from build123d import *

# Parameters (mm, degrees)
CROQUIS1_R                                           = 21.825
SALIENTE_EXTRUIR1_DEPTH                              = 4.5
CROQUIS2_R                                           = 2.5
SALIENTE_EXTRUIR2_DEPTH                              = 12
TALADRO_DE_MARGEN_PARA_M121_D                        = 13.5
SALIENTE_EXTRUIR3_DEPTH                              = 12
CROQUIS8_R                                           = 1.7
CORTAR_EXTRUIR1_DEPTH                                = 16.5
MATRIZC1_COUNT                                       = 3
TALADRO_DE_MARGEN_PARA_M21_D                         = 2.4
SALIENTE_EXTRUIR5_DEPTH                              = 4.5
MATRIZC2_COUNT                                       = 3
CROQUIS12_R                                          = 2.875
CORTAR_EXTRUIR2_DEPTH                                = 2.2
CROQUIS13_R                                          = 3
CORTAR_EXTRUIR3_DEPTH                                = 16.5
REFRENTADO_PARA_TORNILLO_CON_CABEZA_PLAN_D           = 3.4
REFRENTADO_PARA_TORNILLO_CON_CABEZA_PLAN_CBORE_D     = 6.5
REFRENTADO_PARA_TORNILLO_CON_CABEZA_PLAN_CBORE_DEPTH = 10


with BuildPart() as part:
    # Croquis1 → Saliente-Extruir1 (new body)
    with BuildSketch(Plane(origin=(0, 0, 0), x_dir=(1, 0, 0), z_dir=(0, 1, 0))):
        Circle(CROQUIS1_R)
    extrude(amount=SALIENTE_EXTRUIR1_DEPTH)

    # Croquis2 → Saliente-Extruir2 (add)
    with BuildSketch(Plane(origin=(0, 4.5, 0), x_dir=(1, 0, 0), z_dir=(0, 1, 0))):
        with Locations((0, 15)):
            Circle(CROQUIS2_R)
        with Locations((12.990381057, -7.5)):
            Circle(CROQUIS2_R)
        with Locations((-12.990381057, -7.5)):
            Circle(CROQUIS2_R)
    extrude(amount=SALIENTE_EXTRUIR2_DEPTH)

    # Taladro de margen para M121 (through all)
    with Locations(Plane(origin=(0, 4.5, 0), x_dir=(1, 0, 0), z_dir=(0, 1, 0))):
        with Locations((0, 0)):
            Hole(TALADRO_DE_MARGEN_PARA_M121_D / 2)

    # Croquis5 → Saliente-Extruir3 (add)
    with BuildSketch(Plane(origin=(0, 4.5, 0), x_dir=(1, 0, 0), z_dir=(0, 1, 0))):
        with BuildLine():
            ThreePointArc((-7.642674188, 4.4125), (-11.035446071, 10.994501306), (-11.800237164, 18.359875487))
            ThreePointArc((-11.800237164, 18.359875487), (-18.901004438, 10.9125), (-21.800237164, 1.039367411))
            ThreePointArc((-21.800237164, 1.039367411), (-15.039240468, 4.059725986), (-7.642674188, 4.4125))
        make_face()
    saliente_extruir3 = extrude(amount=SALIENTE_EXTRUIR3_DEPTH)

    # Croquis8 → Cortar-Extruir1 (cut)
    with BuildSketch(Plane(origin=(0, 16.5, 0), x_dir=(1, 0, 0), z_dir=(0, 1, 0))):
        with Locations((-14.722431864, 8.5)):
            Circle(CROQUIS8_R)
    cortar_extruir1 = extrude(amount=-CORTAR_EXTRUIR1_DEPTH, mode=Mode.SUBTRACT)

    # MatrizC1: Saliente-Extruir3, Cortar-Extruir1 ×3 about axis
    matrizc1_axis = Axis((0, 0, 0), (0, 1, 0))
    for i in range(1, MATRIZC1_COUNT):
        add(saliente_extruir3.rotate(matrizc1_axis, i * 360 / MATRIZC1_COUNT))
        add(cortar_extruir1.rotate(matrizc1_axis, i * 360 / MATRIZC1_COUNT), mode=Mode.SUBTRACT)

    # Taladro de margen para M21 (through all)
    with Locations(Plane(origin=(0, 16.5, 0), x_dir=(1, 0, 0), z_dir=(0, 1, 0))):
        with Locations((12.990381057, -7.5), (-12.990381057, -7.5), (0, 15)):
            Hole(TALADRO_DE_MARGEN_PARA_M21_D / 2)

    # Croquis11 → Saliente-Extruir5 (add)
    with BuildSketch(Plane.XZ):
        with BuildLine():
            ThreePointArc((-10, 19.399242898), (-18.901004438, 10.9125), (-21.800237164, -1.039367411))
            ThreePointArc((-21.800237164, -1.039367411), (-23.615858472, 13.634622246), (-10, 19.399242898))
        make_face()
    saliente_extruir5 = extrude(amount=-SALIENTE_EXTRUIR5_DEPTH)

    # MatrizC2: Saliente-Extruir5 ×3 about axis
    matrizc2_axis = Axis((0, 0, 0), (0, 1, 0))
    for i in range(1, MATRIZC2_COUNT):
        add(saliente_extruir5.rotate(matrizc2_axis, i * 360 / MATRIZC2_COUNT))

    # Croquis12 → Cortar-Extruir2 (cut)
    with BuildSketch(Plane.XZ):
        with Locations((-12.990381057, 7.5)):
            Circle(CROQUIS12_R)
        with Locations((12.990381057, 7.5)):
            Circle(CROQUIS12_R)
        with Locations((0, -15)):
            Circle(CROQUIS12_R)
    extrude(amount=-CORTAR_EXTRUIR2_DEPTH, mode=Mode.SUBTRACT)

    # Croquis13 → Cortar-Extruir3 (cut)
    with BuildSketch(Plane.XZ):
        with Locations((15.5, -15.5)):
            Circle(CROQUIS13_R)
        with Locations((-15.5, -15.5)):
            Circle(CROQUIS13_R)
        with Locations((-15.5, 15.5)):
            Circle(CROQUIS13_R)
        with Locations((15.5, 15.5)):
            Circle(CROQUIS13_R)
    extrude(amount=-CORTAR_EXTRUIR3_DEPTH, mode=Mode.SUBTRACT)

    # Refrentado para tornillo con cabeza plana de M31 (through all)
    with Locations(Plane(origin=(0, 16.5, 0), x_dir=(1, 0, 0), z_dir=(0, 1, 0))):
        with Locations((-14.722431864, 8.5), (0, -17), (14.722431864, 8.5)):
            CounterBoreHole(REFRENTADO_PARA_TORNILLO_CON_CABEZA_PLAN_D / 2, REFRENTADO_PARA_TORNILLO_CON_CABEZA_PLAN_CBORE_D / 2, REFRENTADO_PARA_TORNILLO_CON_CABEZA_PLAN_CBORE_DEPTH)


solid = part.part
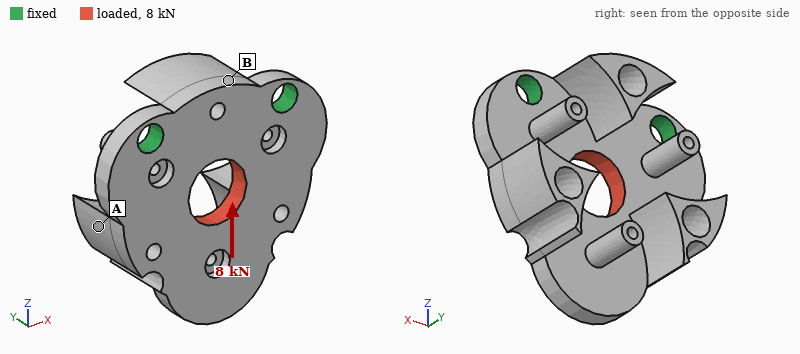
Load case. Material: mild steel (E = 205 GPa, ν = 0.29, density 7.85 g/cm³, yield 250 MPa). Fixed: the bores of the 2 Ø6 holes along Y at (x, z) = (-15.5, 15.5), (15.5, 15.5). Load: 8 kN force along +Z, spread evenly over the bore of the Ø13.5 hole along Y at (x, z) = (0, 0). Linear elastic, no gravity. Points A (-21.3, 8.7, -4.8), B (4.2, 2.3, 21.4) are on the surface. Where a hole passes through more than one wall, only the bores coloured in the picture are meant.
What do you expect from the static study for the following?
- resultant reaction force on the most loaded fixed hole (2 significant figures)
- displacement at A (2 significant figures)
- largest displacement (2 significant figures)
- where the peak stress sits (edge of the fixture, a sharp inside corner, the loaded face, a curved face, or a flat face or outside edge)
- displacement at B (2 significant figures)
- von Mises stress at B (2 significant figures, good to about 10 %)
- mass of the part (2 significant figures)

4.1 kN
3.0 µm
15 µm
a curved face
4.3 µm
39 MPa
78 g
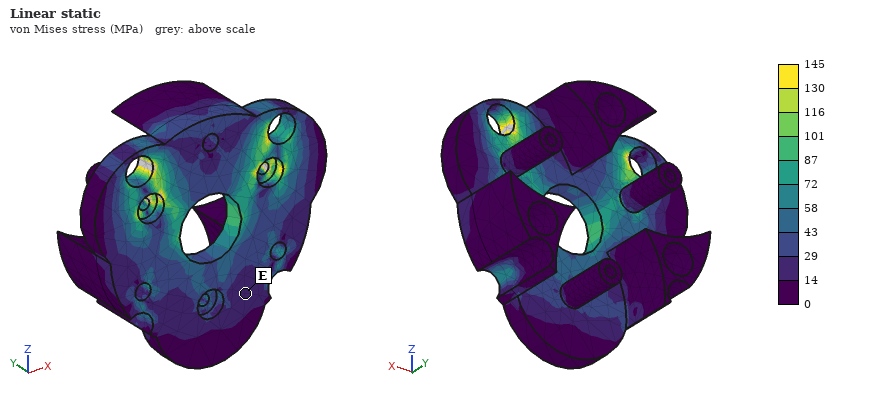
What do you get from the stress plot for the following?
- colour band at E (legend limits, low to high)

14 to 29 MPa
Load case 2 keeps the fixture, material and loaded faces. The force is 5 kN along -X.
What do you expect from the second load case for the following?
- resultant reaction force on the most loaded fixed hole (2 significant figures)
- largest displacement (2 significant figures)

3.2 kN
15 µm
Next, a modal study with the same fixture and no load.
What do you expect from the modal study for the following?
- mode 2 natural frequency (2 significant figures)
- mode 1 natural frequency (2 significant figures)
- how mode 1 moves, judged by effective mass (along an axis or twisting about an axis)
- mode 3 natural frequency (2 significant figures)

5600 Hz
2300 Hz
along Y
10 kHz
